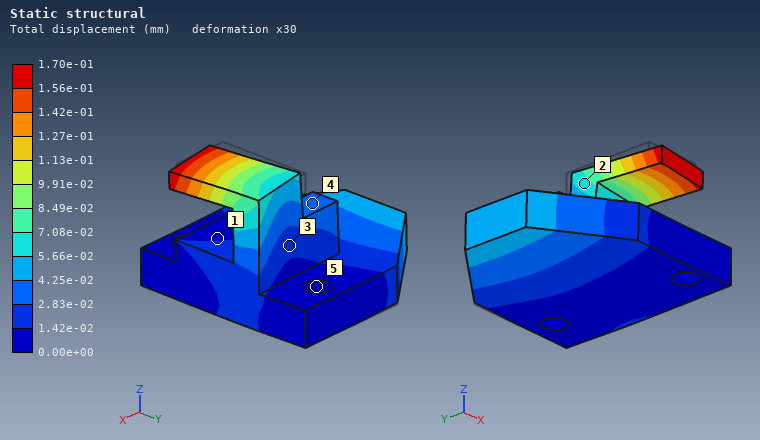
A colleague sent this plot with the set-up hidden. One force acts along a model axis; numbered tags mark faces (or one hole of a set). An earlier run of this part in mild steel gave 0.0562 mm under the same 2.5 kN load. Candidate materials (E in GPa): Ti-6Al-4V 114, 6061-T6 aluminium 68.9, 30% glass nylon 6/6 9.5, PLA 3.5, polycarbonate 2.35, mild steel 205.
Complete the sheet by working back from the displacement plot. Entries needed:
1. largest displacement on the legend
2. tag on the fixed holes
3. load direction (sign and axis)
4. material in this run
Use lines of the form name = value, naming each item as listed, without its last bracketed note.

largest displacement on the legend = 1.70e-01 mm
tag on the fixed holes = 5
load direction = +X
material in this run = 6061-T6 aluminium
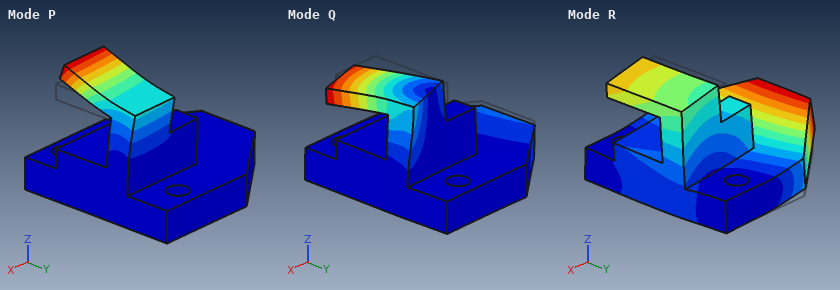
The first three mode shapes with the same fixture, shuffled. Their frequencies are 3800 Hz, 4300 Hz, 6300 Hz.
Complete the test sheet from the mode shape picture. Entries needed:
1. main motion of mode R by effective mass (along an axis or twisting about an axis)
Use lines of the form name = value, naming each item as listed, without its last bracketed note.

main motion of mode R by effective mass = along Z
